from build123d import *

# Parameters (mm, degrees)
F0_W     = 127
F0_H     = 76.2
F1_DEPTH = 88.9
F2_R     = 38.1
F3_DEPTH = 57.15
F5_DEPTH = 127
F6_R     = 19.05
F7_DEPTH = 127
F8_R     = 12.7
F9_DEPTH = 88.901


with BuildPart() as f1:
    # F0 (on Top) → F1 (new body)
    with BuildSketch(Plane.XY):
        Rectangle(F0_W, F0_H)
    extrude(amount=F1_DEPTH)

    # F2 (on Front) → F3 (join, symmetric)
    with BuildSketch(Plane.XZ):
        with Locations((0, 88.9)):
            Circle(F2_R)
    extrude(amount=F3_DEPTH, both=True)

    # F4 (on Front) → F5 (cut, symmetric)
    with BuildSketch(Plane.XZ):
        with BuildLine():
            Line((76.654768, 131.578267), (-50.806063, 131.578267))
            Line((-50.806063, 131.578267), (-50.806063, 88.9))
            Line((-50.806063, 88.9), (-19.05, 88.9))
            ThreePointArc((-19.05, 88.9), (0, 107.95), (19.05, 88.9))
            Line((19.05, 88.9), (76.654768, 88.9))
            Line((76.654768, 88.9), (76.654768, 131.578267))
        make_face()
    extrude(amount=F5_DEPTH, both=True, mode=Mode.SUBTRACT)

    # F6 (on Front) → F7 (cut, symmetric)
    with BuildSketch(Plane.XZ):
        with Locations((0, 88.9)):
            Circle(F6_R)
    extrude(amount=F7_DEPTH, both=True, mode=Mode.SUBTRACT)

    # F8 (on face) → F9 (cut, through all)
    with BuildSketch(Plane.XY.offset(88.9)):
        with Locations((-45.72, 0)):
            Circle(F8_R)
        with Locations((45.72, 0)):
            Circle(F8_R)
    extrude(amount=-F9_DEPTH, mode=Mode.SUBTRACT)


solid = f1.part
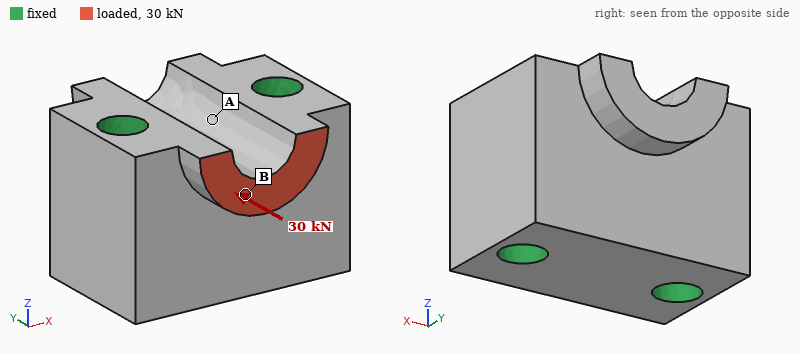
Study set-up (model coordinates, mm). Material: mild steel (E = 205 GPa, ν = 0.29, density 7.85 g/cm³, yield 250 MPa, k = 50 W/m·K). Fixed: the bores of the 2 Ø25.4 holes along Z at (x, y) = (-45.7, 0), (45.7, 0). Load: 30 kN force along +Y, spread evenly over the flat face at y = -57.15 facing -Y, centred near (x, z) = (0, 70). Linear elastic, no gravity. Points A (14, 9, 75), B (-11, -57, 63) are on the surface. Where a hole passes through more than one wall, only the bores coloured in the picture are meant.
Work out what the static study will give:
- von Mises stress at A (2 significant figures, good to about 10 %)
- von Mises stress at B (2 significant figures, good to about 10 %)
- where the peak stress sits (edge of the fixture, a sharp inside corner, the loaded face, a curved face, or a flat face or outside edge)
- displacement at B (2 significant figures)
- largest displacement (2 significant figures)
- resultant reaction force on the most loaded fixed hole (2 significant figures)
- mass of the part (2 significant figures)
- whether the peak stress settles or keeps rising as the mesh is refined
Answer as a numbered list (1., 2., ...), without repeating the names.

1. 4.1 MPa
2. 16 MPa
3. a sharp inside corner
4. 3.9 µm
5. 5.5 µm
6. 16 kN
7. 6.2 kg
8. keeps rising
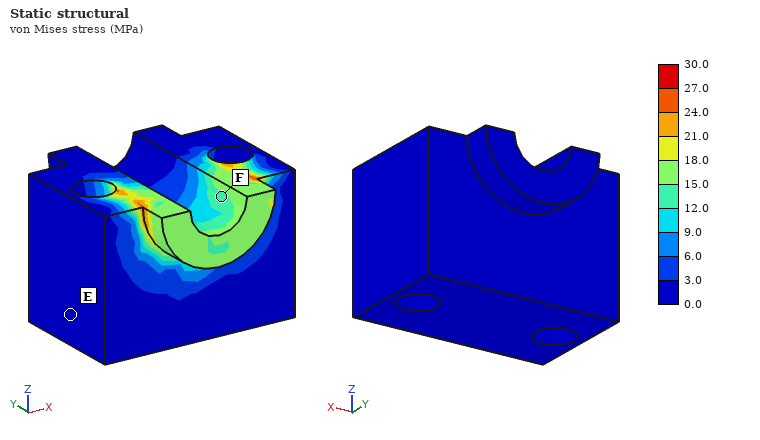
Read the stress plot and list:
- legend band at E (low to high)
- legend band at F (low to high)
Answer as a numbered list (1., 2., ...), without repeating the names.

1. 0.0 to 3.0 MPa
2. 12.0 to 15.0 MPa
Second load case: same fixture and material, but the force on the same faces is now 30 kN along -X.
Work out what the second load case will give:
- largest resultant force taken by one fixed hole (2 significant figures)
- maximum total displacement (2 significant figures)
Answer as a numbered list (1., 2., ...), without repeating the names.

1. 22 kN
2. 20 µm
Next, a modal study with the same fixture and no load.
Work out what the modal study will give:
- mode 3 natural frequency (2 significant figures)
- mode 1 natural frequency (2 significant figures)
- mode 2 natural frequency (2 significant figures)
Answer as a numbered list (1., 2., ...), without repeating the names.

1. 16 kHz
2. 14 kHz
3. 14 kHz
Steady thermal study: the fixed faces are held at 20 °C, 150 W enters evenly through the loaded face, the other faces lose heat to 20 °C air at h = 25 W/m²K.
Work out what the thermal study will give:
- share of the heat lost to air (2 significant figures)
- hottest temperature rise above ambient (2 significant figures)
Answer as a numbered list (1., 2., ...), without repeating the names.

1. 5.5 %
2. 62 K
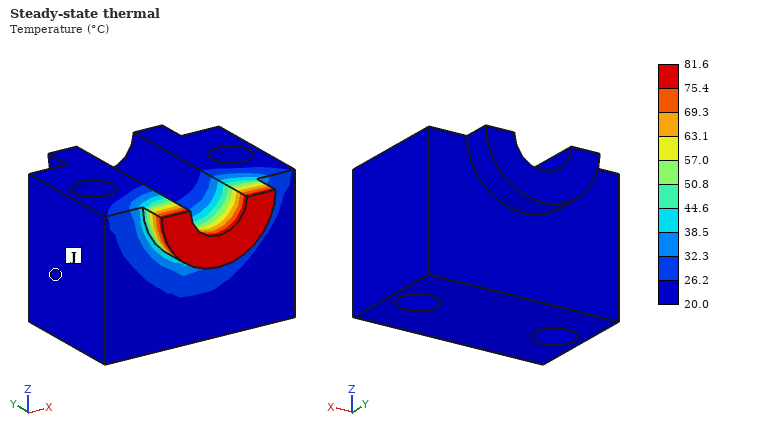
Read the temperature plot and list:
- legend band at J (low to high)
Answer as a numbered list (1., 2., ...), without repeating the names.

1. 20.0 to 26.2 °C
